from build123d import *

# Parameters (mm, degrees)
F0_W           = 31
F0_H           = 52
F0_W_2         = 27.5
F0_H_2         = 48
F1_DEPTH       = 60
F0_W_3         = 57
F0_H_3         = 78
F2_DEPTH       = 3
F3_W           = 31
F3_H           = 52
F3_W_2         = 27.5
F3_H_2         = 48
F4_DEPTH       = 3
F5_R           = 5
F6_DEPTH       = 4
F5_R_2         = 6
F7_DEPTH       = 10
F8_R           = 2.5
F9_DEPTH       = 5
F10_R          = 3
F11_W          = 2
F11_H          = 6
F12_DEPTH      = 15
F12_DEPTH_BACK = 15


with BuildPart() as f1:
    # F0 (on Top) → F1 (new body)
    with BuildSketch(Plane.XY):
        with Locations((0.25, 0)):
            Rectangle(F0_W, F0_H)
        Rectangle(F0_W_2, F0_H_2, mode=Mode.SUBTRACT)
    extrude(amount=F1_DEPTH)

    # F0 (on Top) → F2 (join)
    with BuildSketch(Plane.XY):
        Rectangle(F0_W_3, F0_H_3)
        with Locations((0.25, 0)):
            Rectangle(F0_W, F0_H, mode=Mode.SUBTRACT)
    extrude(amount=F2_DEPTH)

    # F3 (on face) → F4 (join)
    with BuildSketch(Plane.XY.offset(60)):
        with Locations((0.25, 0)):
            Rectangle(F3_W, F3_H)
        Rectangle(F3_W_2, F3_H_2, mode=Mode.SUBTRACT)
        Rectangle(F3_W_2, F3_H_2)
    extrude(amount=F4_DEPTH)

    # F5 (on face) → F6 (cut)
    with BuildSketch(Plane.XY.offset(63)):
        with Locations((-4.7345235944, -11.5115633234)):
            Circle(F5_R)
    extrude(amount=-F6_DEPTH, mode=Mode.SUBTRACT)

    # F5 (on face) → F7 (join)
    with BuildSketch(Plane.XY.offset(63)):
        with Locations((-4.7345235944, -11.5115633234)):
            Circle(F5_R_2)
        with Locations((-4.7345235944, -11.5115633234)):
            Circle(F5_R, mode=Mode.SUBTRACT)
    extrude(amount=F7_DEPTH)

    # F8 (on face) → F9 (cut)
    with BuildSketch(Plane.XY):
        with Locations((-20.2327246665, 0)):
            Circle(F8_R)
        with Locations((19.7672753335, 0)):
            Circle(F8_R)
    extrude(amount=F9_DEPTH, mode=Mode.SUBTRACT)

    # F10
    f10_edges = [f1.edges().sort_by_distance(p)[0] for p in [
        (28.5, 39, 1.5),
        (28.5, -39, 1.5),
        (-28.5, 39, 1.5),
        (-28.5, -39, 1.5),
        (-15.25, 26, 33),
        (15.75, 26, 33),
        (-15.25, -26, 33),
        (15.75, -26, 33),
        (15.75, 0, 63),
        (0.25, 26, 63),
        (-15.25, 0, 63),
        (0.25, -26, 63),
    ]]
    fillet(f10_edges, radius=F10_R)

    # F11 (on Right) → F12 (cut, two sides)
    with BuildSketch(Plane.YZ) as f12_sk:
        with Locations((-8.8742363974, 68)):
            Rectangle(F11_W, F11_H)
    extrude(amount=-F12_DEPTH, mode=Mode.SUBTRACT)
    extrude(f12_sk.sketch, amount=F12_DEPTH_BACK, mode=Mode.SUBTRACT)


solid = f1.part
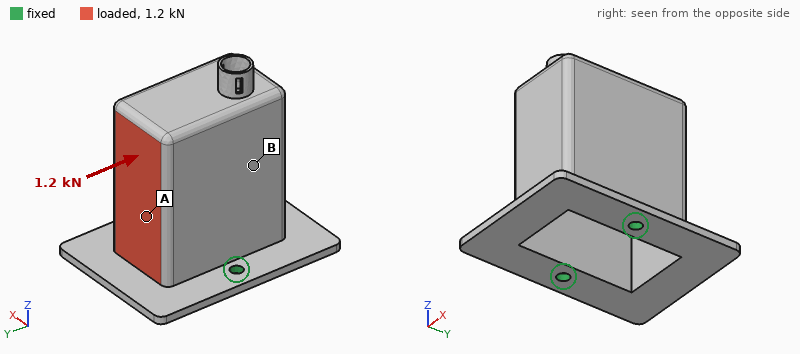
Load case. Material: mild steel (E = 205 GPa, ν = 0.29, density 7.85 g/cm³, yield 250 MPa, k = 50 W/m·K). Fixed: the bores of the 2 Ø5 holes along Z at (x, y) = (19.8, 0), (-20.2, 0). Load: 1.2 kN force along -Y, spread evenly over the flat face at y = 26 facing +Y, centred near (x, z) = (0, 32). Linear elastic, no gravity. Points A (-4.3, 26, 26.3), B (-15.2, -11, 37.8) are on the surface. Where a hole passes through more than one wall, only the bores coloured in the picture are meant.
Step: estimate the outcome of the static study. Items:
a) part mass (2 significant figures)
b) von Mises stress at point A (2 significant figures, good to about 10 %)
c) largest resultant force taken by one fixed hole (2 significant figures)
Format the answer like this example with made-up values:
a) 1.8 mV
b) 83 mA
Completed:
a) 240 g
b) 60 MPa
c) 640 N
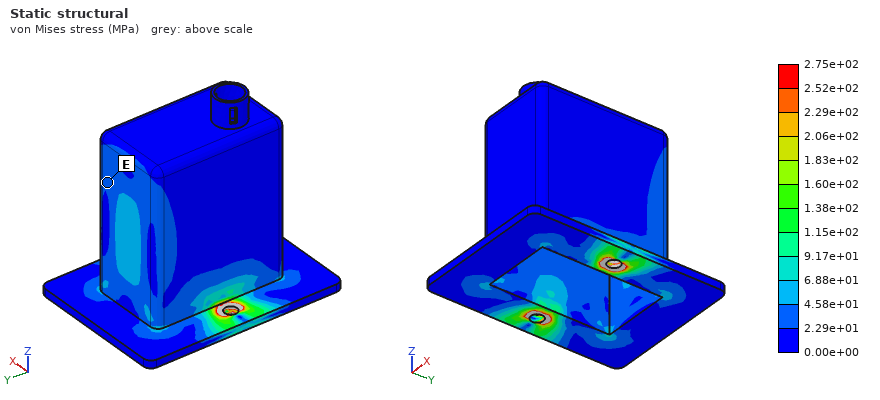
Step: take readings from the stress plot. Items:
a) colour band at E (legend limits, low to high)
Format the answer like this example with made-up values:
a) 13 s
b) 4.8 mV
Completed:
a) 2.29e+01 to 4.58e+01 MPa
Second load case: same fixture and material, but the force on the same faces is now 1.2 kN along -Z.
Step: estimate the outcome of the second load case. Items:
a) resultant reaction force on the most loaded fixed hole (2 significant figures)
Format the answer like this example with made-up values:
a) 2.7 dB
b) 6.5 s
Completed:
a) 610 N
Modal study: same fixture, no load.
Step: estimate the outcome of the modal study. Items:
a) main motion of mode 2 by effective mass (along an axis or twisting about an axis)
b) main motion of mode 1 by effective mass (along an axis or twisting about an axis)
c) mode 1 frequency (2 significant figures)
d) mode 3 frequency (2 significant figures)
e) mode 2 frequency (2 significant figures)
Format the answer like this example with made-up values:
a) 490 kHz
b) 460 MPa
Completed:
a) along X
b) along Y
c) 770 Hz
d) 4000 Hz
e) 2100 Hz
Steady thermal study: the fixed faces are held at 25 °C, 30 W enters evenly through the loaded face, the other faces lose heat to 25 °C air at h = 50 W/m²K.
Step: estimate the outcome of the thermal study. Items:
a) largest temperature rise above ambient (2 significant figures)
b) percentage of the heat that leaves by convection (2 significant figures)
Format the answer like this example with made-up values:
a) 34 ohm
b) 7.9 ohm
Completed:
a) 60 K
b) 78 %
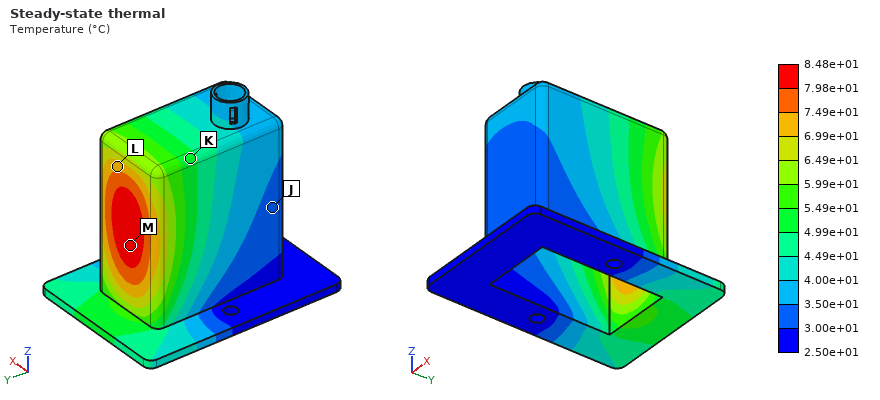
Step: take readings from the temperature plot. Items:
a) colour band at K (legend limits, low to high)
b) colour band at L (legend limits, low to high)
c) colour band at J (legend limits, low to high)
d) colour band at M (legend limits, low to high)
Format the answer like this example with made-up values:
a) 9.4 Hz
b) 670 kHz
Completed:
a) 4.99e+01 to 5.49e+01 °C
b) 6.99e+01 to 7.49e+01 °C
c) 3.00e+01 to 3.50e+01 °C
d) 7.98e+01 to 8.48e+01 °C
